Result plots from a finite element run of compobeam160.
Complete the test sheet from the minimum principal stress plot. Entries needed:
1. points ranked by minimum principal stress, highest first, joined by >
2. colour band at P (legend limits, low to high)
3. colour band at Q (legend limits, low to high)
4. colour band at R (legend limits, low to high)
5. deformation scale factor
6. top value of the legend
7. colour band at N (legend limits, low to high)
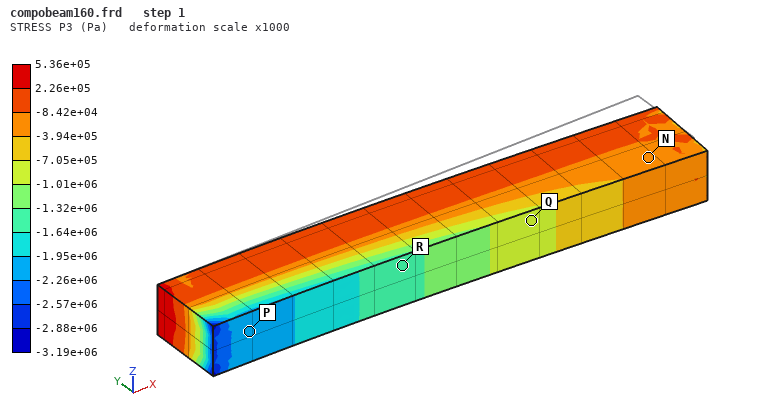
N > Q > R > P
-2.26e+06 to -1.95e+06 Pa
-1.01e+06 to -7.05e+05 Pa
-1.64e+06 to -1.32e+06 Pa
1000
5.36e+05 Pa
-3.94e+05 to -8.42e+04 Pa
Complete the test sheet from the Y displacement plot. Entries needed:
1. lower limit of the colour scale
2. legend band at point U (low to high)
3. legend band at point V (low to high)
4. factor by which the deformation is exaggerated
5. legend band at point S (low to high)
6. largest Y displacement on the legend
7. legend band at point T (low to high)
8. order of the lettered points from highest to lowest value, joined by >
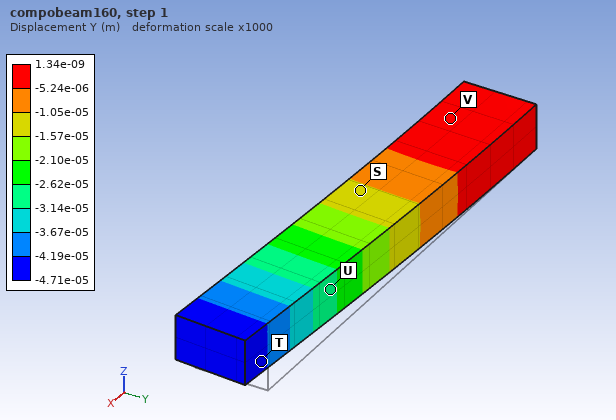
-4.71e-05 m
-3.14e-05 to -2.62e-05 m
-5.24e-06 to 1.34e-09 m
1000
-1.57e-05 to -1.05e-05 m
1.34e-09 m
-4.71e-05 to -4.19e-05 m
V > S > U > T
